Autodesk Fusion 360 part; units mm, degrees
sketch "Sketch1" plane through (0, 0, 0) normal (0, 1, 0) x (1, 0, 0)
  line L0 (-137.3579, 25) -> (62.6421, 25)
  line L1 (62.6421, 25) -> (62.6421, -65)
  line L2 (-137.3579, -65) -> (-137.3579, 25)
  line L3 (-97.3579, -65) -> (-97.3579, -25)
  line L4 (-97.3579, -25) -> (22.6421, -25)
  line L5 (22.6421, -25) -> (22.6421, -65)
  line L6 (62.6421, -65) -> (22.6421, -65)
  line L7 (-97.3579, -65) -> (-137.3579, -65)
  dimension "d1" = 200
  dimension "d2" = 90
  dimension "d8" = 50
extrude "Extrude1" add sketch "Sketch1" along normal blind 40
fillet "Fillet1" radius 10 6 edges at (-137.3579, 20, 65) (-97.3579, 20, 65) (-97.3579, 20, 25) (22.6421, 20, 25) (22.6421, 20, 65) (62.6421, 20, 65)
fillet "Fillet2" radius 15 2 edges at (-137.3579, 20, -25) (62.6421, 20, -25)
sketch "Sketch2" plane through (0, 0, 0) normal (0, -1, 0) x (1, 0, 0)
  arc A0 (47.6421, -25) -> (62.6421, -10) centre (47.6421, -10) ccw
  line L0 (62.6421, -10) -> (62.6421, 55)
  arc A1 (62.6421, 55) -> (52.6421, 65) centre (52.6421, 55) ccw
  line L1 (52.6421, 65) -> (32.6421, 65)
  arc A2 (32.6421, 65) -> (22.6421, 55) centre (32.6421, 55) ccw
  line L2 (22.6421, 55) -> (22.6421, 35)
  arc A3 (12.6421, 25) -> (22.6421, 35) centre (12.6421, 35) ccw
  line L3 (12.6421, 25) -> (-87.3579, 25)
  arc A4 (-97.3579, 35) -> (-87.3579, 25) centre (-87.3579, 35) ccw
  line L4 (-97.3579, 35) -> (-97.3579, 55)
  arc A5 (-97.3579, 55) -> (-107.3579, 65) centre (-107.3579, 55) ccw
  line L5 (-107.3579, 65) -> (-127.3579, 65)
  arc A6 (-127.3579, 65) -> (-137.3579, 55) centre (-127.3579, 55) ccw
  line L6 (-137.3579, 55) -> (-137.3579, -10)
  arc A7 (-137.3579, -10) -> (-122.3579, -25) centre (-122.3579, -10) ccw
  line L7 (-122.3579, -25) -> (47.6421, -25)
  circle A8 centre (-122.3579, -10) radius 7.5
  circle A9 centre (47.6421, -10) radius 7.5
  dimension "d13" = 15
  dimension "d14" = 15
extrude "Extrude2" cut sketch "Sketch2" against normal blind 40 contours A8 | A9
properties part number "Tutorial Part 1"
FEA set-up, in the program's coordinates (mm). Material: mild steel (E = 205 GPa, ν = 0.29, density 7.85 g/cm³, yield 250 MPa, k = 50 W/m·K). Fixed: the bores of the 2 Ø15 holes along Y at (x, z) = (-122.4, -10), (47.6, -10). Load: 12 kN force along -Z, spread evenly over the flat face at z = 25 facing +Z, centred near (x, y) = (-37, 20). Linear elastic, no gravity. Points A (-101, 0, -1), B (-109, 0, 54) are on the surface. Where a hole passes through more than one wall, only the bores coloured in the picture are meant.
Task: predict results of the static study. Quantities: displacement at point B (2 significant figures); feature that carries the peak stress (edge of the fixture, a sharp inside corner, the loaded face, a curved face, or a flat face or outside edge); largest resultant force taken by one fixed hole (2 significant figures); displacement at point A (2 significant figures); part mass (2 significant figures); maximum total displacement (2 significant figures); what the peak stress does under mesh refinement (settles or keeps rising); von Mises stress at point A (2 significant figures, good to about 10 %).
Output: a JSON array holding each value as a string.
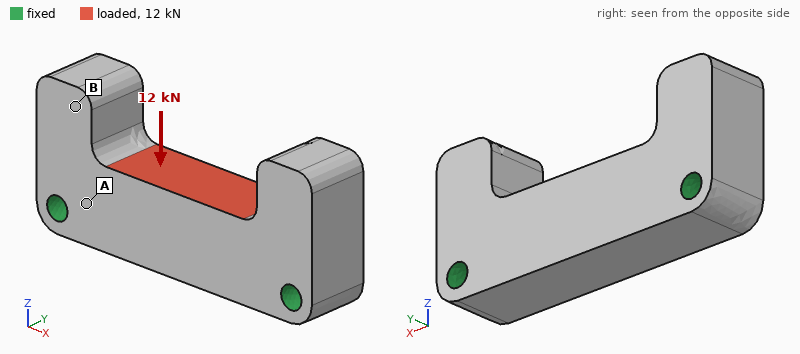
["5.0 µm", "edge of the fixture", "7.1 kN", "2.0 µm", "4.0 kg", "7.1 µm", "keeps rising", "7.9 MPa"]
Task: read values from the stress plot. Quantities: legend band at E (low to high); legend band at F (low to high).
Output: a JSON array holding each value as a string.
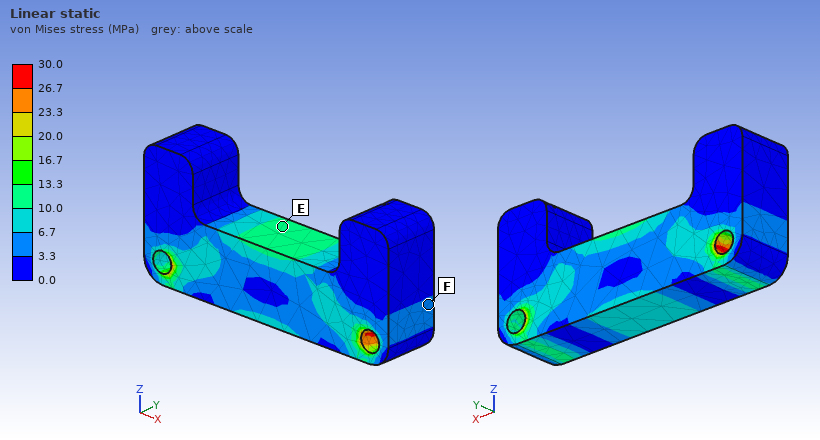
["10.0 to 13.3 MPa", "3.3 to 6.7 MPa"]
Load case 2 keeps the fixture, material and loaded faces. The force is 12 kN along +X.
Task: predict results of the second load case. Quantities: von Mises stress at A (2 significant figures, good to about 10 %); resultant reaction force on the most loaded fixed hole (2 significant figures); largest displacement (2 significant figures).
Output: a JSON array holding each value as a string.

["4.7 MPa", "6.4 kN", "1.7 µm"]
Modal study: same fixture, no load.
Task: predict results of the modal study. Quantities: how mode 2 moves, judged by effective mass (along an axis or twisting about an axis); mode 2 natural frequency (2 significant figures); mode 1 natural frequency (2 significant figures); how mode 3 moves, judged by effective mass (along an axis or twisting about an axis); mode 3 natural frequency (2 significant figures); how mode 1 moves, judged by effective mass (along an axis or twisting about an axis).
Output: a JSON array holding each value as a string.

["along Y", "4700 Hz", "4400 Hz", "twisting about Z", "5600 Hz", "along Z"]
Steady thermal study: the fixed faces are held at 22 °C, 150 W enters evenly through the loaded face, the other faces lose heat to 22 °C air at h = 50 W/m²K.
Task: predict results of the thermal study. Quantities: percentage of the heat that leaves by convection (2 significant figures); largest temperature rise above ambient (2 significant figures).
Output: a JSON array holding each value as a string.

["23 %", "49 K"]
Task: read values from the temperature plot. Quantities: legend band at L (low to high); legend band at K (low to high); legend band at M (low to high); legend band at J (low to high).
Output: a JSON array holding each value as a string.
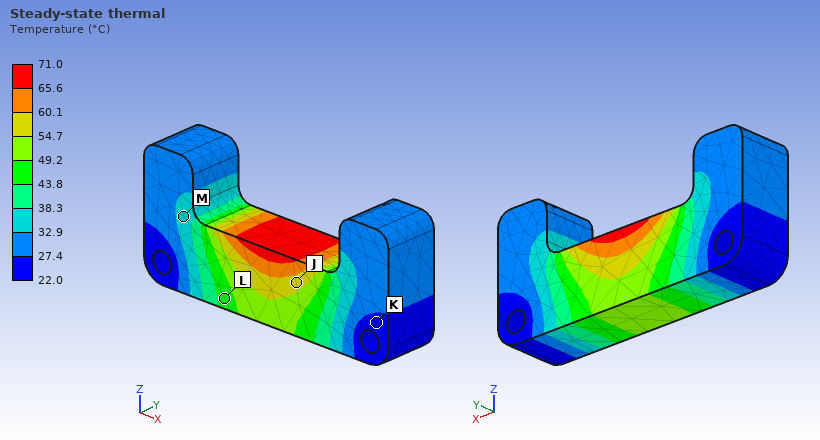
["43.8 to 49.2 °C", "22.0 to 27.4 °C", "32.9 to 38.3 °C", "54.7 to 60.1 °C"]
